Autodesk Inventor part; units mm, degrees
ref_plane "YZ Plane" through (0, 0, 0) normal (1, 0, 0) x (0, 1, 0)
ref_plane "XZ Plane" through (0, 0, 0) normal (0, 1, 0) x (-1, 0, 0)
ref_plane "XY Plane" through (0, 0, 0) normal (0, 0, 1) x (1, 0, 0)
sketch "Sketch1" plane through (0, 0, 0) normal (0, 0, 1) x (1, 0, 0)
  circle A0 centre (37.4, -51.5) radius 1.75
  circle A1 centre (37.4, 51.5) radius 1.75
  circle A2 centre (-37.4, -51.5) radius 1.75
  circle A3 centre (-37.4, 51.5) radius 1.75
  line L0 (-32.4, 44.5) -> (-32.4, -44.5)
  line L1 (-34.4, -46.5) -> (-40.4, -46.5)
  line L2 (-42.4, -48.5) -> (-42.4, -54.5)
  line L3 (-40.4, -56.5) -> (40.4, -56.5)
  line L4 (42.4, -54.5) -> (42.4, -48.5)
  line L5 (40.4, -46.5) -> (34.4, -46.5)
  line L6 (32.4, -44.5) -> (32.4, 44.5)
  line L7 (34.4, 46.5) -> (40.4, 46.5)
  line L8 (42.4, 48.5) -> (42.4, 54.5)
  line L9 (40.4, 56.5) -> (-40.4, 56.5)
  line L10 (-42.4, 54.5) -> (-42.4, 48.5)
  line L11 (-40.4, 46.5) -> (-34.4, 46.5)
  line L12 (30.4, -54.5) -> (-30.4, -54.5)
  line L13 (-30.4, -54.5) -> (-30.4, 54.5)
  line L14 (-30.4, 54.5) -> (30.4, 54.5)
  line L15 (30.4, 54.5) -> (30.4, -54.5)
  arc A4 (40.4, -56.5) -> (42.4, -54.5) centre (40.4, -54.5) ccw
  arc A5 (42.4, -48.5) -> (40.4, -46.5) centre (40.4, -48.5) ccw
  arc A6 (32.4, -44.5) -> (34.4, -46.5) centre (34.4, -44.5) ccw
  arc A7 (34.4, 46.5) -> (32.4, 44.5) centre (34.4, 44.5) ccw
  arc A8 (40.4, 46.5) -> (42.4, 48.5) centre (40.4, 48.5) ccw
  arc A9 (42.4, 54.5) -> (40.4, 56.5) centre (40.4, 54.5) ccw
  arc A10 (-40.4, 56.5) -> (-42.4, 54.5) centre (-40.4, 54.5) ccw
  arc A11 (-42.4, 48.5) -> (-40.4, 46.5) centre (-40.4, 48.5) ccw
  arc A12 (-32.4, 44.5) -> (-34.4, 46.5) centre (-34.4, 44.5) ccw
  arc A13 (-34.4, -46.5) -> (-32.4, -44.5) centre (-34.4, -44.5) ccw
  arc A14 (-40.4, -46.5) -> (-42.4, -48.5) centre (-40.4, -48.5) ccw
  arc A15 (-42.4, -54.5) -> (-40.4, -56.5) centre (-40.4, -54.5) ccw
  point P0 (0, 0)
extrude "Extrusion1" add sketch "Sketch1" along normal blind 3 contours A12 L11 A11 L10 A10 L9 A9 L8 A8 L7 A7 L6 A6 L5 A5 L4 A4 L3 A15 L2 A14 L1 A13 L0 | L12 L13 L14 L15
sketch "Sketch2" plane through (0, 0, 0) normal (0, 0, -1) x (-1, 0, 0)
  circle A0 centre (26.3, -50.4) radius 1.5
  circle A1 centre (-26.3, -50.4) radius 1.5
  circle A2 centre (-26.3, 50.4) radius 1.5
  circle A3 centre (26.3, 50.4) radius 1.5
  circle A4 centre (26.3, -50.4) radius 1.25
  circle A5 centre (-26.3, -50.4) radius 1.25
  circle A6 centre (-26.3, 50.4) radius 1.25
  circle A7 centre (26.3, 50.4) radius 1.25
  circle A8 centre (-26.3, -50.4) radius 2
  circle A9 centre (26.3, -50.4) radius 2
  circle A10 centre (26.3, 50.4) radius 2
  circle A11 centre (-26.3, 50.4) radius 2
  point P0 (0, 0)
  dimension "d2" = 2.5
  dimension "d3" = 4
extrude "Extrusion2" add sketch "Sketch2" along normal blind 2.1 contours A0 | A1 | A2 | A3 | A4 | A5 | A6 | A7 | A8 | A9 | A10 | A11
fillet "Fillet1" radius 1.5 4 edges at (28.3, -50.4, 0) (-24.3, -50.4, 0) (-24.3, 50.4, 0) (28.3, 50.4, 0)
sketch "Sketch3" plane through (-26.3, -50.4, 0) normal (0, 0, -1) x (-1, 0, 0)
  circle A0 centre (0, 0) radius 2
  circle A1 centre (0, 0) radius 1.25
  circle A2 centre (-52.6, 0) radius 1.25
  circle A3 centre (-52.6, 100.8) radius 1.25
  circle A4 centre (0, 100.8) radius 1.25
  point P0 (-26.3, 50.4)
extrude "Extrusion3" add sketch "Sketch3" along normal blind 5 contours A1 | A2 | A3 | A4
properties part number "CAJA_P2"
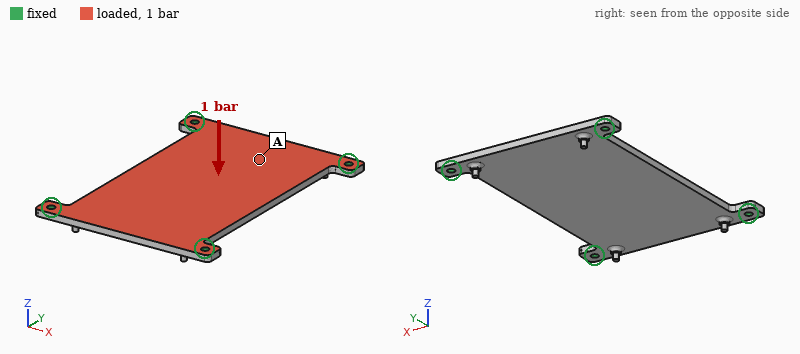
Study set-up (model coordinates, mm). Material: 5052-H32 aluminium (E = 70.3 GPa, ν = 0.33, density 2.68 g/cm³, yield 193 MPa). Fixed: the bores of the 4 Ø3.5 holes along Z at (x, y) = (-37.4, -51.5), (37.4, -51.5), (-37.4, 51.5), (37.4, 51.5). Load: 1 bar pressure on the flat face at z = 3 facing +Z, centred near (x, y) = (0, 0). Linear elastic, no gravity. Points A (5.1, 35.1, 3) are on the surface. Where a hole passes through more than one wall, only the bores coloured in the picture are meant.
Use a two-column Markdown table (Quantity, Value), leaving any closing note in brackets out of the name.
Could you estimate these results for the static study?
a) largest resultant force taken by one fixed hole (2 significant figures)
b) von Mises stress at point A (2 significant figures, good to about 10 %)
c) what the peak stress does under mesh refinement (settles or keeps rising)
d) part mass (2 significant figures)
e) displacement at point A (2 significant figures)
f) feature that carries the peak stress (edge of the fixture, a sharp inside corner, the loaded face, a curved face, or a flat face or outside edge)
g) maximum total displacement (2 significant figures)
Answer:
| Quantity | Value |
|---|---|
| largest resultant force taken by one fixed hole | 190 N |
| von Mises stress at point A | 23 MPa |
| what the peak stress does under mesh refinement | keeps rising |
| part mass | 62 g |
| displacement at point A | 0.23 mm |
| feature that carries the peak stress | edge of the fixture |
| maximum total displacement | 0.42 mm |
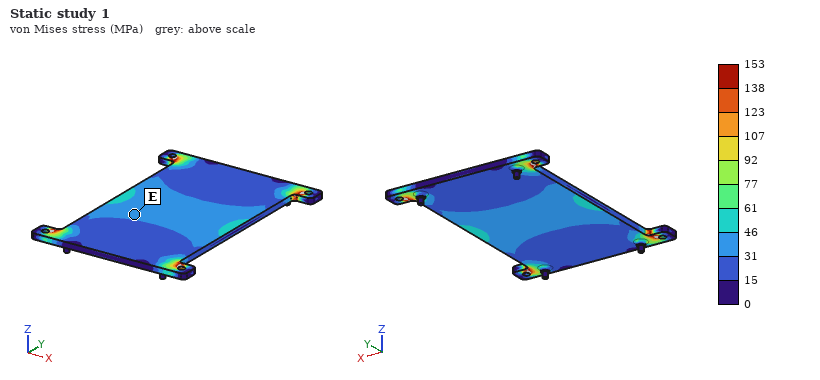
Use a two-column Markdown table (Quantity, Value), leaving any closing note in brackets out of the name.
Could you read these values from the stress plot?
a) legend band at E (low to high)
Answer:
| Quantity | Value |
|---|---|
| legend band at E | 31 to 46 MPa |
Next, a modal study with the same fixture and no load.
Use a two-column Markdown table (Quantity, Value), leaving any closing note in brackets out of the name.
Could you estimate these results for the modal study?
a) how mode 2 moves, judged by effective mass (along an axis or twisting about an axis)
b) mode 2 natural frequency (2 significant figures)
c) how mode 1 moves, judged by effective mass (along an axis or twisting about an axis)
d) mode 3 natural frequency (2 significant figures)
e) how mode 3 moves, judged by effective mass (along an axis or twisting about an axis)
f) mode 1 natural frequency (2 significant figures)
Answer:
| Quantity | Value |
|---|---|
| how mode 2 moves, judged by effective mass | twisting about Y |
| mode 2 natural frequency | 2000 Hz |
| how mode 1 moves, judged by effective mass | along Z |
| mode 3 natural frequency | 2400 Hz |
| how mode 3 moves, judged by effective mass | twisting about X |
| mode 1 natural frequency | 990 Hz |
